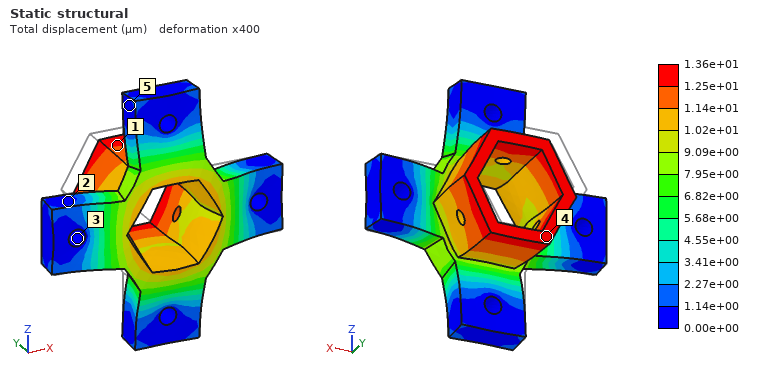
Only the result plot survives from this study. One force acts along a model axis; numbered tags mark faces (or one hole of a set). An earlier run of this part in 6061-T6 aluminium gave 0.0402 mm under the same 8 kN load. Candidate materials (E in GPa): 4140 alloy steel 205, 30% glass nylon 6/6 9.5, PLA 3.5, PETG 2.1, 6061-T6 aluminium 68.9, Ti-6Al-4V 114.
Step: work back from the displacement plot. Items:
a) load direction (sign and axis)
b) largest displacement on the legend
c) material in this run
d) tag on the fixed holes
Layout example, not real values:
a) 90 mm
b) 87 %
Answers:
a) -Y
b) 1.36e+01 µm
c) 4140 alloy steel
d) 3
